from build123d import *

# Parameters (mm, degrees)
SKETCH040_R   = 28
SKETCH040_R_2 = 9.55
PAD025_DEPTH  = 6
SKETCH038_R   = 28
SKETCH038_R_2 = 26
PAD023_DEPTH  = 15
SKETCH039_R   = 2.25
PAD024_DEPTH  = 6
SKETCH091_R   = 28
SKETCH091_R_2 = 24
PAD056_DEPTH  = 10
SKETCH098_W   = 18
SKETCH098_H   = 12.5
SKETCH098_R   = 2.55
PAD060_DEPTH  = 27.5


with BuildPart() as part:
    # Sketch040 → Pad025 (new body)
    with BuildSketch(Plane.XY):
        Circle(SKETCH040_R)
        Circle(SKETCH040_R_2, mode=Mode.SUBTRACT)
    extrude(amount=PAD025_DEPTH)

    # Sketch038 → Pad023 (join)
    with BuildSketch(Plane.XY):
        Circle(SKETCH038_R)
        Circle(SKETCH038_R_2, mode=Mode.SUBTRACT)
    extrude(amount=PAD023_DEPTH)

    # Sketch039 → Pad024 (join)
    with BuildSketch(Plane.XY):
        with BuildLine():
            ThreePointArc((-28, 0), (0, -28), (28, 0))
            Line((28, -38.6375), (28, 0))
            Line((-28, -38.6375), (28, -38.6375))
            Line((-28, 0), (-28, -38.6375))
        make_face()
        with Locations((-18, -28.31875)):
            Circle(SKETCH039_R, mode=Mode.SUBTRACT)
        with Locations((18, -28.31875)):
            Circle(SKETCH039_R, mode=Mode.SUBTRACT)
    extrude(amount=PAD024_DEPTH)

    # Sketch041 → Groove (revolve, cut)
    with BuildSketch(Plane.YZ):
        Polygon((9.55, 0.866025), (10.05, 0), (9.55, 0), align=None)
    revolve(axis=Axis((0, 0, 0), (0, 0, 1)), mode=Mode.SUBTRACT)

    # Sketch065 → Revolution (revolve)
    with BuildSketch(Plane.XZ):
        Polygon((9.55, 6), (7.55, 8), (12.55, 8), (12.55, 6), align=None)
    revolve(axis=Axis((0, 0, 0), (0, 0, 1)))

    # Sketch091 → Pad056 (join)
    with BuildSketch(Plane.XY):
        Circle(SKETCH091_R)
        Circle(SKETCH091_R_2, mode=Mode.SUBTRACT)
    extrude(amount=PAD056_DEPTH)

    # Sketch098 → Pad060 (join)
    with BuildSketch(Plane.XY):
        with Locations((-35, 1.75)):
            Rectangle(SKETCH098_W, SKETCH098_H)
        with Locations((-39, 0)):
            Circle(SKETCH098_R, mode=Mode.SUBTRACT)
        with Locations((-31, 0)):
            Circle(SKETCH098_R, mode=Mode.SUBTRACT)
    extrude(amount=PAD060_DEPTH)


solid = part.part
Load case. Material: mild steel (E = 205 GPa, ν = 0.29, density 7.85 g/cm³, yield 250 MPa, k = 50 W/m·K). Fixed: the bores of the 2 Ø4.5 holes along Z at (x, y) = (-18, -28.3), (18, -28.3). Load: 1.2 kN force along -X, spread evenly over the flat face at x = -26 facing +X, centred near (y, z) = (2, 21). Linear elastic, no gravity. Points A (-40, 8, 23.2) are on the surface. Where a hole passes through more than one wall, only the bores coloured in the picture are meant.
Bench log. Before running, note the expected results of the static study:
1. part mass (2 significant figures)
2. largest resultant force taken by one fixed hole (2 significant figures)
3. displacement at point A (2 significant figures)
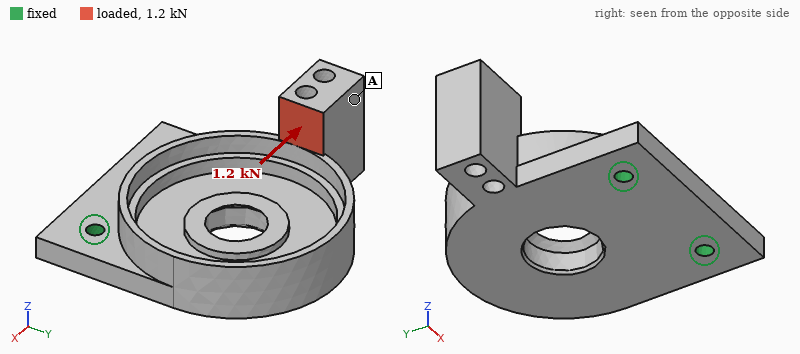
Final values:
220 g
1.3 kN
0.092 mm
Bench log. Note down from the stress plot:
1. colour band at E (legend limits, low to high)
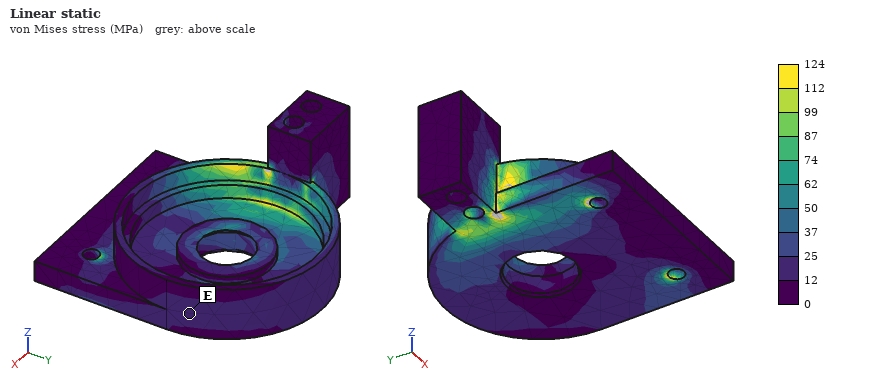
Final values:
12 to 25 MPa
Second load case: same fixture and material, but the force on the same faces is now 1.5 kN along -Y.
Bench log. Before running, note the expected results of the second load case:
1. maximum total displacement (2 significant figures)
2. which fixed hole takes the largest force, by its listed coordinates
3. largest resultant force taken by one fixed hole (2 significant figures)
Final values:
0.13 mm
(-18, -28.3)
1.8 kN
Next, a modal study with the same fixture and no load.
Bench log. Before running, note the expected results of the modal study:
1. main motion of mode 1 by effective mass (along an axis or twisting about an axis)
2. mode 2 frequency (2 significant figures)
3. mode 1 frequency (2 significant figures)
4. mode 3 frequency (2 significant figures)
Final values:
along Z
2700 Hz
1500 Hz
5600 Hz
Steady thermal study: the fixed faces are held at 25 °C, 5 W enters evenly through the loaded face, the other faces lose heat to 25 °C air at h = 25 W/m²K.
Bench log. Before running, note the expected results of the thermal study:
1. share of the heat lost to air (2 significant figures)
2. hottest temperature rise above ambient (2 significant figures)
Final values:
40 %
24 K
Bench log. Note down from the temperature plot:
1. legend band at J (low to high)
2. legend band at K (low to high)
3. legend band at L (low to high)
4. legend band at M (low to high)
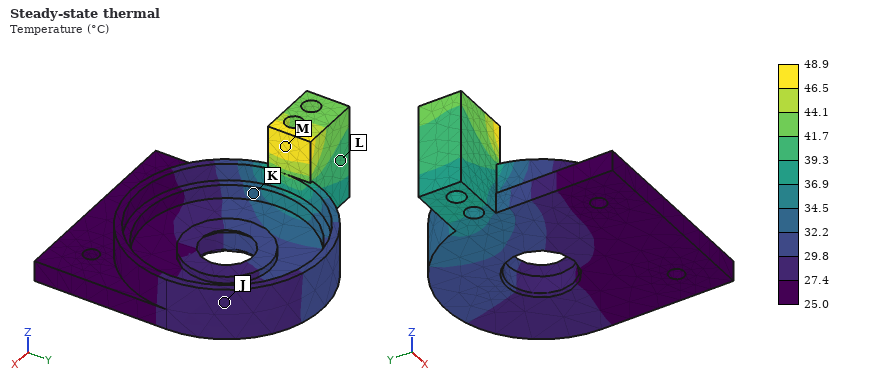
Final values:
27.4 to 29.8 °C
32.2 to 34.5 °C
39.3 to 41.7 °C
46.5 to 48.9 °C
